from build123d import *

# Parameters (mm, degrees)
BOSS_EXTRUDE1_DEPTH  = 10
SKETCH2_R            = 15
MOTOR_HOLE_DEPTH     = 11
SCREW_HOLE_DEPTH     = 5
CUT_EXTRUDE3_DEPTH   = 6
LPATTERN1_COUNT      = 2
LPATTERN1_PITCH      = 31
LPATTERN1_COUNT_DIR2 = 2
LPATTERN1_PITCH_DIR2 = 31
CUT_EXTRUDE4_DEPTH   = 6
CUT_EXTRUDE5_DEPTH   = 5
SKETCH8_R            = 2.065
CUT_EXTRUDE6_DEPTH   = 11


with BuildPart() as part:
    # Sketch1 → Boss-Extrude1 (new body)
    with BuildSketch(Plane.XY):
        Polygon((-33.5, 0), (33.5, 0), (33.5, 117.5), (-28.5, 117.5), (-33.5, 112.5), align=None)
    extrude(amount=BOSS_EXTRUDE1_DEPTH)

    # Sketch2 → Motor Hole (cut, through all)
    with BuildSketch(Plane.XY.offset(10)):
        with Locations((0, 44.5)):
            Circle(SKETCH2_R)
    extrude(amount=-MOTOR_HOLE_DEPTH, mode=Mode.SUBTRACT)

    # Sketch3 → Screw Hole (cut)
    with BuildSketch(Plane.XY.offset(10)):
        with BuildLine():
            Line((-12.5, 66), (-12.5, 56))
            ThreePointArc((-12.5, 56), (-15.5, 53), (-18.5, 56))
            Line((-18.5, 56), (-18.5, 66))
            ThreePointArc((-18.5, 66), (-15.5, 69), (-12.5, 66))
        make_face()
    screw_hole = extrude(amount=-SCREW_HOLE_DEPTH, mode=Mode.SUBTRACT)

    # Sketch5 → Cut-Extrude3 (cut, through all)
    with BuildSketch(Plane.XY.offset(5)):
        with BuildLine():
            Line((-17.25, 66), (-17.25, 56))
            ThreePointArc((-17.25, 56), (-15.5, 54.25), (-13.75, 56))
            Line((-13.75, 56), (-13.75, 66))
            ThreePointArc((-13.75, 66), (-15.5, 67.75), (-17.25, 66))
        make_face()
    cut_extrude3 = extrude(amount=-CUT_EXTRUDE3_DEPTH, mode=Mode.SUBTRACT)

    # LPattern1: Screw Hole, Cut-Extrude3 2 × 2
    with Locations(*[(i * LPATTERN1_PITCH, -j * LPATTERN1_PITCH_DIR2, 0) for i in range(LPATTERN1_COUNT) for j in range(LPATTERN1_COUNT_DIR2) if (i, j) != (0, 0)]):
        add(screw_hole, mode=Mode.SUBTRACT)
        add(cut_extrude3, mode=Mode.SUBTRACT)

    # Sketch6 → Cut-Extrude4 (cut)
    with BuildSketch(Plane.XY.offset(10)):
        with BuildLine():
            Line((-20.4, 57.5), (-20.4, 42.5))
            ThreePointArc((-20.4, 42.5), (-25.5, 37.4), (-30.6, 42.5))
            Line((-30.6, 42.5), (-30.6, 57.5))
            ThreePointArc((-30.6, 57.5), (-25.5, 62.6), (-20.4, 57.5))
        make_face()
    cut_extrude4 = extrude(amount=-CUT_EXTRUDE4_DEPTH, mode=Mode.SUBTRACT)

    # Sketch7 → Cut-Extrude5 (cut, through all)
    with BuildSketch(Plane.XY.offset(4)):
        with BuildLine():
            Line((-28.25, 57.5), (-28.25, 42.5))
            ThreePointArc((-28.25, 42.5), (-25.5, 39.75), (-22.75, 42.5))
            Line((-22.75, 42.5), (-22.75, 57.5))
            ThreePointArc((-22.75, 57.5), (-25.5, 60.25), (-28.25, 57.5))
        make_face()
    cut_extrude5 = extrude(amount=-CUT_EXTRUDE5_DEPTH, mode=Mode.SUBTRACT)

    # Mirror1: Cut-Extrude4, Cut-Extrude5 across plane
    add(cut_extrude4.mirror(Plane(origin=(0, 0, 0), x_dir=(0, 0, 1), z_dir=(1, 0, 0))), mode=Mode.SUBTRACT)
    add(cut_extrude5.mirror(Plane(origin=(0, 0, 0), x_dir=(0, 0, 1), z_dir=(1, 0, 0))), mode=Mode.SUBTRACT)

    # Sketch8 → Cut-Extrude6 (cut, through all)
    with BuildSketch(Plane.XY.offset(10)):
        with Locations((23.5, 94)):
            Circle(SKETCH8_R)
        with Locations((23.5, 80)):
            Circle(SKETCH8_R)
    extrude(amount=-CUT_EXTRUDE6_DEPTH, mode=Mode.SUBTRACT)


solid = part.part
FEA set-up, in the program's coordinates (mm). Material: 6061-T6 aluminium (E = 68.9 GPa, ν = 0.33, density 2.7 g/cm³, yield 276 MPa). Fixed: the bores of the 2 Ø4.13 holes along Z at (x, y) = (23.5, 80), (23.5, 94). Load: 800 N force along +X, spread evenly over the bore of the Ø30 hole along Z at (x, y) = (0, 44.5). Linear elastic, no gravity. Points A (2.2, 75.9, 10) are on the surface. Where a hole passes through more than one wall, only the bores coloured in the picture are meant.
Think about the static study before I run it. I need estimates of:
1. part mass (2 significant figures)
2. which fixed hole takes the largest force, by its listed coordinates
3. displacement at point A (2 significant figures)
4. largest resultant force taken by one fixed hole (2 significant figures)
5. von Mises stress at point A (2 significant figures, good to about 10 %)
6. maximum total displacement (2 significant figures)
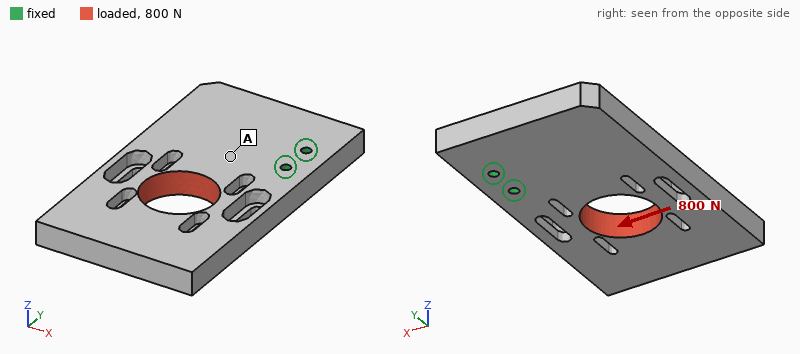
180 g
(23.5, 80)
8.0 µm
2.3 kN
5.0 MPa
49 µm
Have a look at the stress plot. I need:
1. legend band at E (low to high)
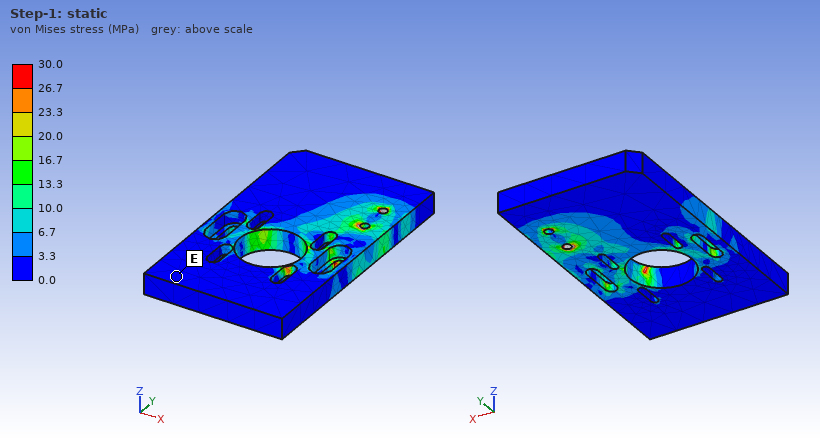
0.0 to 3.3 MPa
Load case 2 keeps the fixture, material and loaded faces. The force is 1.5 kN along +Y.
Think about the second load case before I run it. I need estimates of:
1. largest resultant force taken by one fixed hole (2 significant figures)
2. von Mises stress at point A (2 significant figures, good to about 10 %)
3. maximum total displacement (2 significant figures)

2.2 kN
5.6 MPa
42 µm
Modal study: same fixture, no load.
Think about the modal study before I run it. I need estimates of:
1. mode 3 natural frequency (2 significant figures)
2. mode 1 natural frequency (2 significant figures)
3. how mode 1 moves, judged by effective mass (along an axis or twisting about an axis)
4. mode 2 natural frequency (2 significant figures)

1900 Hz
780 Hz
along Z
1700 Hz
